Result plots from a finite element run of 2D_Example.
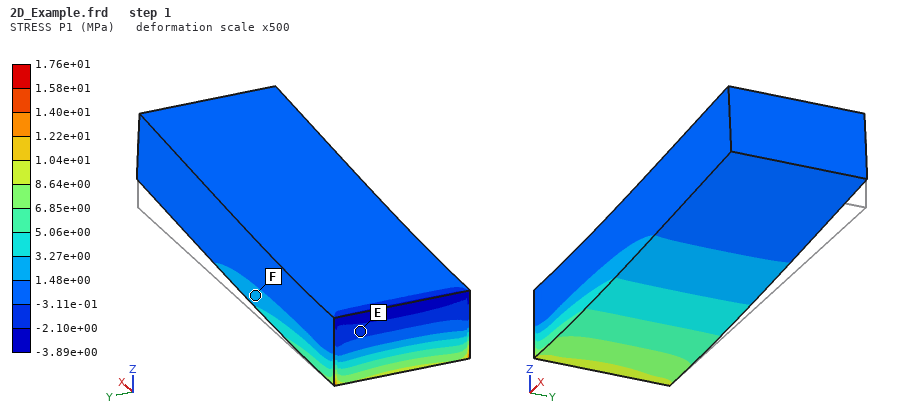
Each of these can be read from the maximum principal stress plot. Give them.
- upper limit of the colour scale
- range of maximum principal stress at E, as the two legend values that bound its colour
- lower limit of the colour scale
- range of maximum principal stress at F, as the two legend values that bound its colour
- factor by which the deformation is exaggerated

1.76e+01 MPa
-2.10e+00 to -3.11e-01 MPa
-3.89e+00 MPa
1.48e+00 to 3.27e+00 MPa
500
